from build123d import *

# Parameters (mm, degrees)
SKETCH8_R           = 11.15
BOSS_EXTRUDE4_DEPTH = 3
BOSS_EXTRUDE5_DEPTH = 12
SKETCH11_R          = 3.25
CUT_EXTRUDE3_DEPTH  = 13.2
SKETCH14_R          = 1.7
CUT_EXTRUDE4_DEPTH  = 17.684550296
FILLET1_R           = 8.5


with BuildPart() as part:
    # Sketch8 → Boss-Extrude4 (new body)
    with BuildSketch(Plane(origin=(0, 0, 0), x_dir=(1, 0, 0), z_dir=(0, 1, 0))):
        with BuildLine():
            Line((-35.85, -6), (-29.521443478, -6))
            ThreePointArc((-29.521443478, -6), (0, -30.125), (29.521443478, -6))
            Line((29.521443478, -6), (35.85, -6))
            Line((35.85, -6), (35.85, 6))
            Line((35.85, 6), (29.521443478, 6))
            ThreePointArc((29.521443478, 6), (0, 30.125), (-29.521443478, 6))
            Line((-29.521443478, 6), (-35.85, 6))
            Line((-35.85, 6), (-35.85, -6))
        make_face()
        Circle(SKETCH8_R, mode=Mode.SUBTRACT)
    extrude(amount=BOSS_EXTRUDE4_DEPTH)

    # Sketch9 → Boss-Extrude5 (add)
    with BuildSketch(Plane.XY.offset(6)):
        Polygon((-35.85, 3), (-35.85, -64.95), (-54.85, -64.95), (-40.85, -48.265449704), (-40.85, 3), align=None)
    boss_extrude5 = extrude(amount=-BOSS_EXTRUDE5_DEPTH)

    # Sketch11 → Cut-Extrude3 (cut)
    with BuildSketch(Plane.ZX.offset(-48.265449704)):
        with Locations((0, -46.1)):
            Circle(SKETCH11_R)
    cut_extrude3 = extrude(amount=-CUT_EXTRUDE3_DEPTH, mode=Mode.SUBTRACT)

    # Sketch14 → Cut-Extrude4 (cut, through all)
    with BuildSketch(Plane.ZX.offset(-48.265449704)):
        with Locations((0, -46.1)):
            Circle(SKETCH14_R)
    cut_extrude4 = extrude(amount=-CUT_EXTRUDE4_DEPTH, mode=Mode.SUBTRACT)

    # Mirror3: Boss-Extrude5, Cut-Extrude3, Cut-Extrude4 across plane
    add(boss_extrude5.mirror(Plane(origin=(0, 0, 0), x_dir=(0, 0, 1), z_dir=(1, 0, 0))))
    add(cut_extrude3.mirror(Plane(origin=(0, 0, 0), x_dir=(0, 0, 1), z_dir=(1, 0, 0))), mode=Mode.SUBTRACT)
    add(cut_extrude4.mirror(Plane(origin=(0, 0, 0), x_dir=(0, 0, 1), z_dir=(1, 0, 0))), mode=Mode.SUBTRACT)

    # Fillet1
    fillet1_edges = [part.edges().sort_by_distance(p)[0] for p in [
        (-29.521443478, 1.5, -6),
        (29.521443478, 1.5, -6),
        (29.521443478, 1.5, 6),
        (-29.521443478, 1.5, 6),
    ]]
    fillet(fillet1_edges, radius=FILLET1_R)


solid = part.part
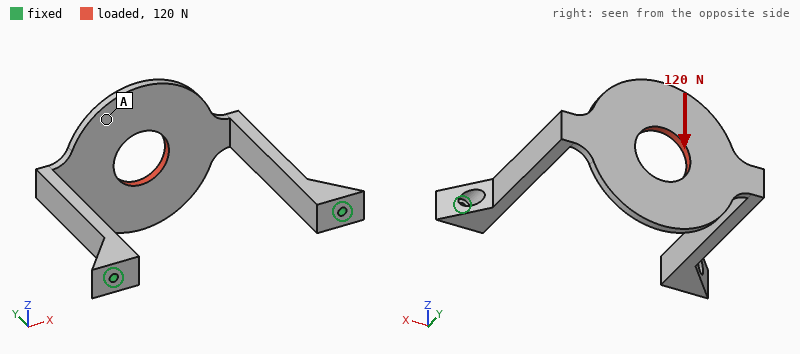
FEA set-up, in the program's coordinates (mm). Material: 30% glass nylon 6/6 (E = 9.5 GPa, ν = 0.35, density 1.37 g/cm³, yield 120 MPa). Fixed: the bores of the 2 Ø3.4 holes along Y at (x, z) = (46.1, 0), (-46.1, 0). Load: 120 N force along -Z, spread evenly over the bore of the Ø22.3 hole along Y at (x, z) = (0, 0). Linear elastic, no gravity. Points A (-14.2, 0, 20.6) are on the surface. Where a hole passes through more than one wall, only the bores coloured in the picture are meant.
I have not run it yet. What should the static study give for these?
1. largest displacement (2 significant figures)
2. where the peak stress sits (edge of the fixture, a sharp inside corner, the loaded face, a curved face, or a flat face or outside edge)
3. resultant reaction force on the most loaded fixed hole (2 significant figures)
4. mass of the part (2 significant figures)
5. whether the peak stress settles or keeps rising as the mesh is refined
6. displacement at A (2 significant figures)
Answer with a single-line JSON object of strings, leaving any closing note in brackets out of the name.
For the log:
{"largest displacement": "1.7 mm", "where the peak stress sits": "edge of the fixture", "resultant reaction force on the most loaded fixed hole": "60 N", "mass of the part": "25 g", "whether the peak stress settles or keeps rising as the mesh is refined": "keeps rising", "displacement at A": "1.5 mm"}
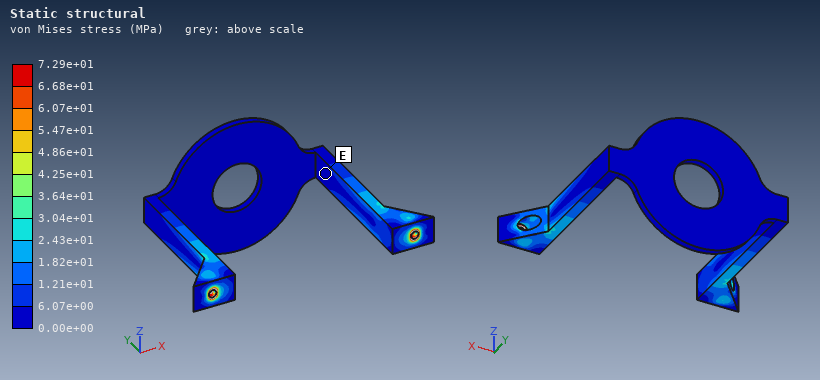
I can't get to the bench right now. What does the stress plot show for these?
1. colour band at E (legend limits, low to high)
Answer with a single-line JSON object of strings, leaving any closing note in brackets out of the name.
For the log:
{"colour band at E": "0.00e+00 to 6.07e+00 MPa"}
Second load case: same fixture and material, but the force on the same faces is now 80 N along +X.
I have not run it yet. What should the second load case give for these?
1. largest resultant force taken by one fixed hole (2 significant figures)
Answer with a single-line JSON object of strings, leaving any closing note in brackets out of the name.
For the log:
{"largest resultant force taken by one fixed hole": "44 N"}
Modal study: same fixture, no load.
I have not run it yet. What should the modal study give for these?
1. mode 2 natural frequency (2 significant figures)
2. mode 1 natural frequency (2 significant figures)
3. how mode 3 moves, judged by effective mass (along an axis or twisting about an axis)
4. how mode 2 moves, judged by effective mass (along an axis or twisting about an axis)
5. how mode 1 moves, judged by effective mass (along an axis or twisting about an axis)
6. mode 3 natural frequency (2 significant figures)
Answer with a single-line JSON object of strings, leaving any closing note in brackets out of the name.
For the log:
{"mode 2 natural frequency": "380 Hz", "mode 1 natural frequency": "340 Hz", "how mode 3 moves, judged by effective mass": "twisting about Y", "how mode 2 moves, judged by effective mass": "along Z", "how mode 1 moves, judged by effective mass": "along X", "mode 3 natural frequency": "660 Hz"}
